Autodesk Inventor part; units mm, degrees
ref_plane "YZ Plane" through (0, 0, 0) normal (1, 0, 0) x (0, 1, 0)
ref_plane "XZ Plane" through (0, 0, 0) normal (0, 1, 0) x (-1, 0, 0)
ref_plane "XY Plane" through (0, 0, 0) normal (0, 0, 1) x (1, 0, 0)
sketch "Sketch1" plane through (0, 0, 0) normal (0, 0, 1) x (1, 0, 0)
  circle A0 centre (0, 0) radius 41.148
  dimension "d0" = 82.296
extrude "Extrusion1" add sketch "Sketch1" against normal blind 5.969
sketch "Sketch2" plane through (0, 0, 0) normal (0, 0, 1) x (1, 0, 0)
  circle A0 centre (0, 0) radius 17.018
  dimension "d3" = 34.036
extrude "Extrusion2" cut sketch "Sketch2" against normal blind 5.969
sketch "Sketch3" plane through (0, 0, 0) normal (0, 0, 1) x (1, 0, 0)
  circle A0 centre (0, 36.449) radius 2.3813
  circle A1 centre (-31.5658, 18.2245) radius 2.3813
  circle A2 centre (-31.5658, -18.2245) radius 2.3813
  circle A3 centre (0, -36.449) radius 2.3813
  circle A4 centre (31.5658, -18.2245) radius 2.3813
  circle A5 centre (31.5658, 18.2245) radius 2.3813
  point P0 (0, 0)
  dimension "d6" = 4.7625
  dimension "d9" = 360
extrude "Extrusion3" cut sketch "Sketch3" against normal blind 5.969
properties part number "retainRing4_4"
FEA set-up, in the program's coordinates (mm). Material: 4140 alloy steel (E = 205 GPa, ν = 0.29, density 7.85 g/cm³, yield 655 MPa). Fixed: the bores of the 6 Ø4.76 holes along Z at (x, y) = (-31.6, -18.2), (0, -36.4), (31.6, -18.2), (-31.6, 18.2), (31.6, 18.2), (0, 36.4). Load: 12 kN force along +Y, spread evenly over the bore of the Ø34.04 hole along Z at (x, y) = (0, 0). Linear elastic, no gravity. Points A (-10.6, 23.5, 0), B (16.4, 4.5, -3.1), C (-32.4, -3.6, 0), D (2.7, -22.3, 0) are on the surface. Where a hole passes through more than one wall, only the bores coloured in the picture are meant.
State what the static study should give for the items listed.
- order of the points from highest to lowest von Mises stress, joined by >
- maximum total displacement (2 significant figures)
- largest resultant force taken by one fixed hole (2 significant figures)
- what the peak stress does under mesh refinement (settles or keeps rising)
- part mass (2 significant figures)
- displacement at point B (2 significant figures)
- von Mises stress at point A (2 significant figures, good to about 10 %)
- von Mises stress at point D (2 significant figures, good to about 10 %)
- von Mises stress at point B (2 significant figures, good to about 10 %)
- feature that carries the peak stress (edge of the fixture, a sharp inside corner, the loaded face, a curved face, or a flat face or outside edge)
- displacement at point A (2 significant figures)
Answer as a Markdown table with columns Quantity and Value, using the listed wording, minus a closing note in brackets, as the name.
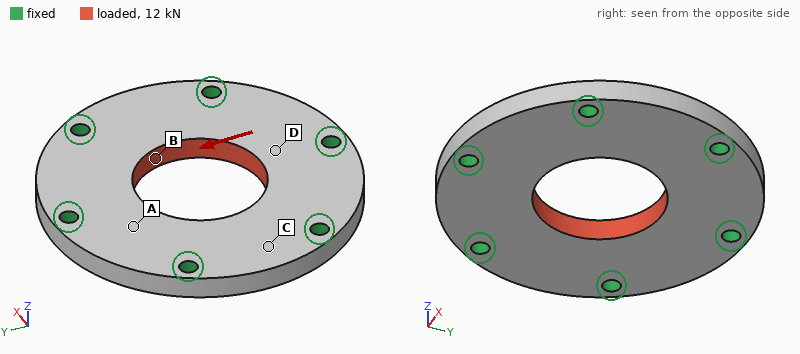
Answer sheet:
| Quantity | Value |
|---|---|
| order of the points from highest to lowest von Mises stress, joined by > | B > D > A > C |
| maximum total displacement | 2.9 µm |
| largest resultant force taken by one fixed hole | 2.8 kN |
| what the peak stress does under mesh refinement | keeps rising |
| part mass | 200 g |
| displacement at point B | 2.7 µm |
| von Mises stress at point A | 15 MPa |
| von Mises stress at point D | 25 MPa |
| von Mises stress at point B | 33 MPa |
| feature that carries the peak stress | edge of the fixture |
| displacement at point A | 2.1 µm |
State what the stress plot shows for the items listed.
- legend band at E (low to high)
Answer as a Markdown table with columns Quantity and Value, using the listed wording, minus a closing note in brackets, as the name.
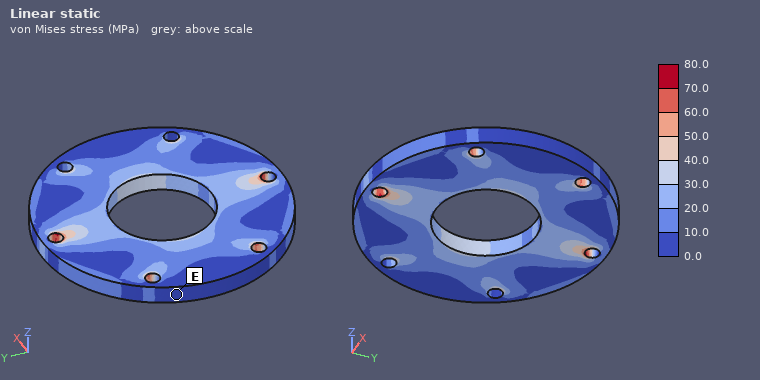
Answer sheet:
| Quantity | Value |
|---|---|
| legend band at E | 0.0 to 10.0 MPa |
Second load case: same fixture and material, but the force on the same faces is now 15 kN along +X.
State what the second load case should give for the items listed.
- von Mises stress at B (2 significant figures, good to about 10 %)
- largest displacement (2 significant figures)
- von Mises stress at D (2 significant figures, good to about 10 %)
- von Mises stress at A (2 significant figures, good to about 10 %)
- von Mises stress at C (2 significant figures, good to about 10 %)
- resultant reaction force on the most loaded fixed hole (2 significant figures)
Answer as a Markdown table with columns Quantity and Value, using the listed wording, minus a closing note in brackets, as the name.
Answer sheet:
| Quantity | Value |
|---|---|
| von Mises stress at B | 22 MPa |
| largest displacement | 3.7 µm |
| von Mises stress at D | 17 MPa |
| von Mises stress at A | 16 MPa |
| von Mises stress at C | 8.6 MPa |
| resultant reaction force on the most loaded fixed hole | 3.1 kN |
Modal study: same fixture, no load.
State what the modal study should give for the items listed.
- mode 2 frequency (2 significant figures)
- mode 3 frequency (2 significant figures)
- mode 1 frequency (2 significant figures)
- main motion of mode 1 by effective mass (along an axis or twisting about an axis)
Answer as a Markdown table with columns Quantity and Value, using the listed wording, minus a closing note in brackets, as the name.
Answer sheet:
| Quantity | Value |
|---|---|
| mode 2 frequency | 16 kHz |
| mode 3 frequency | 16 kHz |
| mode 1 frequency | 13 kHz |
| main motion of mode 1 by effective mass | along Z |
